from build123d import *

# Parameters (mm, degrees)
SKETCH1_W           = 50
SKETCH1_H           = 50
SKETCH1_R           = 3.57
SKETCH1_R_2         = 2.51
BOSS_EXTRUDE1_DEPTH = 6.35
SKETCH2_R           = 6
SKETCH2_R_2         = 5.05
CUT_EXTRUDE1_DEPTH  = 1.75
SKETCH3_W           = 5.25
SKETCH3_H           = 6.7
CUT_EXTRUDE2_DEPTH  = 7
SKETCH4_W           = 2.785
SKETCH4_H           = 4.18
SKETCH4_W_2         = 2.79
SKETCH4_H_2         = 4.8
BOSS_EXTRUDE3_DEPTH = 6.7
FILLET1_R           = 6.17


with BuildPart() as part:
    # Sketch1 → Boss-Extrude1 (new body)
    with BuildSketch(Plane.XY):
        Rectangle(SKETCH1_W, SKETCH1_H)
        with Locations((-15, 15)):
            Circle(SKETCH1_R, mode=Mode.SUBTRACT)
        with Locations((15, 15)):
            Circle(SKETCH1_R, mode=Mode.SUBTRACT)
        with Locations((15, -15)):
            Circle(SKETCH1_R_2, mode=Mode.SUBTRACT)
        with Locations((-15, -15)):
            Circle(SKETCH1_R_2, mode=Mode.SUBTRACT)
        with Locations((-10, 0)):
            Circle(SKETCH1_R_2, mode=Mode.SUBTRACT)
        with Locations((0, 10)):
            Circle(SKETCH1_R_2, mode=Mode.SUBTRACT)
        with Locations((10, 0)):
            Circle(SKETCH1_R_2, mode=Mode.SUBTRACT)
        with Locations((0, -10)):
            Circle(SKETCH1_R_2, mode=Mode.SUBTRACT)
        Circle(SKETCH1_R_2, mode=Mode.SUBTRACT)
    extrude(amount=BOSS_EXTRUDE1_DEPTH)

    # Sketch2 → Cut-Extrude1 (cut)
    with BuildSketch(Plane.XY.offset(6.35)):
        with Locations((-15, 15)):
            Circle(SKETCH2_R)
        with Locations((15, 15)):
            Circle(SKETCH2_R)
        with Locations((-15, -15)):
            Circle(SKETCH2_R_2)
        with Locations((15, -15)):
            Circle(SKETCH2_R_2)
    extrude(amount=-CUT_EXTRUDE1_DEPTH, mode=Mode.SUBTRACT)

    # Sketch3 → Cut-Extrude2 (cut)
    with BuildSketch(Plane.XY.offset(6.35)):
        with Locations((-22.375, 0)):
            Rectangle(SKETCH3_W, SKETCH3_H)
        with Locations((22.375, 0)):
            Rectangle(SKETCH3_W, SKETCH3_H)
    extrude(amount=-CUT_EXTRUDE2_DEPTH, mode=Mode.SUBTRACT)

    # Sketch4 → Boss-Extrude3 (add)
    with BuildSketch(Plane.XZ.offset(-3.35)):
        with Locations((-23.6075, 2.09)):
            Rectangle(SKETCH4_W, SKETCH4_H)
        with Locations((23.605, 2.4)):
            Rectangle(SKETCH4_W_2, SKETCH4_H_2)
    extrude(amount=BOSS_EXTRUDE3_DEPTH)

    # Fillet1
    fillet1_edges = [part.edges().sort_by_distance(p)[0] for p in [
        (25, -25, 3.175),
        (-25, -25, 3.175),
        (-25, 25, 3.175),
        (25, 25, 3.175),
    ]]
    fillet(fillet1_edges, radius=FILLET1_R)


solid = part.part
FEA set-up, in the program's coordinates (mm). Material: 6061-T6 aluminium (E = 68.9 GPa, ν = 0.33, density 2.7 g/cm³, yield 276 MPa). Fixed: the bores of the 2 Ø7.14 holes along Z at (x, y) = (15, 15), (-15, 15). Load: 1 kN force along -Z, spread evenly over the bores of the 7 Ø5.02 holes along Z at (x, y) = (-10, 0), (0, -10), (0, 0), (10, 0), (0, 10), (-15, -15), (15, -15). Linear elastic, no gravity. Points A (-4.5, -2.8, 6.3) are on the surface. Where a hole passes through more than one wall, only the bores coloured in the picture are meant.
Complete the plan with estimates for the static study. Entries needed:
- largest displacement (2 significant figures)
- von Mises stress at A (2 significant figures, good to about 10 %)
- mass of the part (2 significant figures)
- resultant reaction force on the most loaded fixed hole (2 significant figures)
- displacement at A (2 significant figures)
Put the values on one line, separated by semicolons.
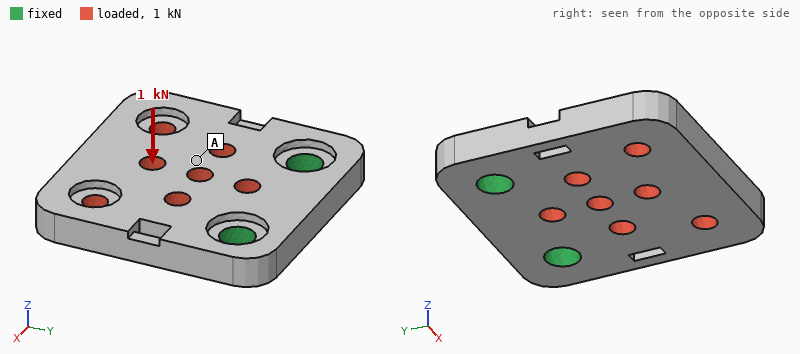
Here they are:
0.13 mm; 17 MPa; 37 g; 510 N; 0.048 mm
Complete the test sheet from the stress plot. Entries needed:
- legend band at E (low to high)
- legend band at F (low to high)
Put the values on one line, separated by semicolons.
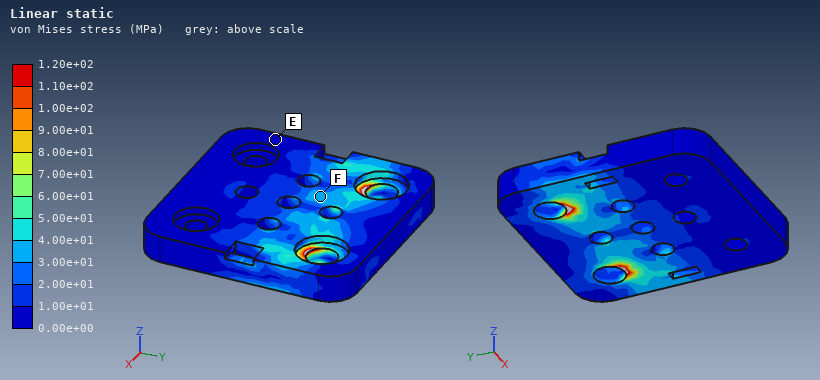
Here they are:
0.00e+00 to 1.00e+01 MPa; 3.00e+01 to 4.00e+01 MPa
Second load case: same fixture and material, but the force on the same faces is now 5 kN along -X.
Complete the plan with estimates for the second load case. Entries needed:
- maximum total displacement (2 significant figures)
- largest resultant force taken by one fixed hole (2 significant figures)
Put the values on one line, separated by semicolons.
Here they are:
34 µm; 3.5 kN
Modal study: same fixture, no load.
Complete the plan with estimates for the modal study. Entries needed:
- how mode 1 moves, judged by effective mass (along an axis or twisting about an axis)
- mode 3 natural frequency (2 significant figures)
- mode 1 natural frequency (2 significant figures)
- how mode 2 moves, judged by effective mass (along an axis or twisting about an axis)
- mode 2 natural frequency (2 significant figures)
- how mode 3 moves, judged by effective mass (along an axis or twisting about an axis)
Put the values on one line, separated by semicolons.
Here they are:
along Z; 12 kHz; 2900 Hz; twisting about Y; 5900 Hz; along X
